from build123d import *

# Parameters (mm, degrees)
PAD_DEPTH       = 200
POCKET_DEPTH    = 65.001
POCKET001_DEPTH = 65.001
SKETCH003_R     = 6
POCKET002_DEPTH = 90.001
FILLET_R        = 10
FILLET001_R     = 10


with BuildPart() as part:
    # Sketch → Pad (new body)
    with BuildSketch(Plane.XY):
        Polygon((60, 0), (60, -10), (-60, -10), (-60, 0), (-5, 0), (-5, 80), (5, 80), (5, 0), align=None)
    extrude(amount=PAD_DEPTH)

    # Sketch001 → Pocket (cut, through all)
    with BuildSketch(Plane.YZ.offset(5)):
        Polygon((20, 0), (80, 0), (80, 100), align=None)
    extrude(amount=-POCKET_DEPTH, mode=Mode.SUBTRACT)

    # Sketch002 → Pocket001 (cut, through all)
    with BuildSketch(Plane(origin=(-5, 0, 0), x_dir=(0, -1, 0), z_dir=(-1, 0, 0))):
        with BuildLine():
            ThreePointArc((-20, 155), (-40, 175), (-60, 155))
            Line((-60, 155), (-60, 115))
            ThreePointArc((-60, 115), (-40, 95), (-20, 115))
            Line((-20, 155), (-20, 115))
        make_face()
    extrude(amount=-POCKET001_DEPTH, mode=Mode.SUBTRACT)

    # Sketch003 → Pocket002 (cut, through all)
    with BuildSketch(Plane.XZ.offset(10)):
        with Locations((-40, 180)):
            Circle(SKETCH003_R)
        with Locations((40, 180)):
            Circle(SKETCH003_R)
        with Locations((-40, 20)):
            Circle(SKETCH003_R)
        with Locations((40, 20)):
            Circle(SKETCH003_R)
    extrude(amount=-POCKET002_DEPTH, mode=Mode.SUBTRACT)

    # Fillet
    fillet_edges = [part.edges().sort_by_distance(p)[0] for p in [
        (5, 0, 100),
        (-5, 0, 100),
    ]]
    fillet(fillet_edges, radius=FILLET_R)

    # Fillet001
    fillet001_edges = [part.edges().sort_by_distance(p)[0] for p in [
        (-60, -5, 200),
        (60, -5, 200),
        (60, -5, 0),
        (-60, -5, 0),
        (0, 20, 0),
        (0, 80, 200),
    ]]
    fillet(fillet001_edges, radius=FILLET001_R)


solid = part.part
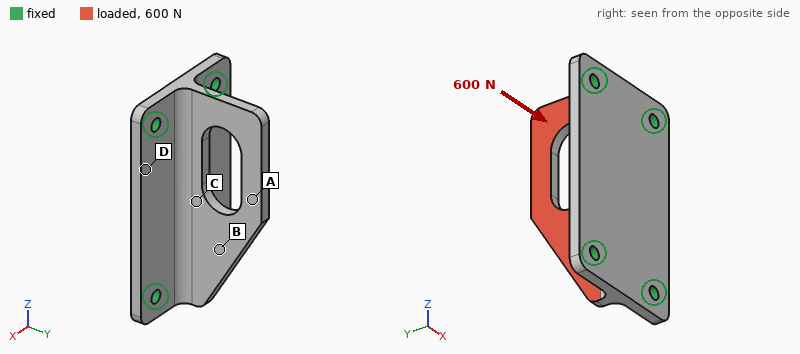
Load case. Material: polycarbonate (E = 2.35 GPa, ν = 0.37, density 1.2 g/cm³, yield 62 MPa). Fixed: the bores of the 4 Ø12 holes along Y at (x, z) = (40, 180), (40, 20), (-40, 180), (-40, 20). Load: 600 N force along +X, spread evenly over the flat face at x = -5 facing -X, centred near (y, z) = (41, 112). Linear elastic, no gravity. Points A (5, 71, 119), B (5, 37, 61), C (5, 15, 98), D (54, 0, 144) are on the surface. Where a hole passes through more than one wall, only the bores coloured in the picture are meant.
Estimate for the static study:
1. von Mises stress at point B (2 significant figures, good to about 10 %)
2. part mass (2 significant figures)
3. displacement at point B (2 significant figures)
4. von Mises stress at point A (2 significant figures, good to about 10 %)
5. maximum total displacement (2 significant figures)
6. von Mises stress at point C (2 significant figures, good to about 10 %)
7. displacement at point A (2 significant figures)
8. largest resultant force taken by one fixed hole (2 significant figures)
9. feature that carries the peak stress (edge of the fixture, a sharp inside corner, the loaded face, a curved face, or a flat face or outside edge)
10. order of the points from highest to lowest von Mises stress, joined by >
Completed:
4.5 MPa
410 g
0.48 mm
2.7 MPa
2.4 mm
6.4 MPa
1.9 mm
310 N
the loaded face
C > B > A > D
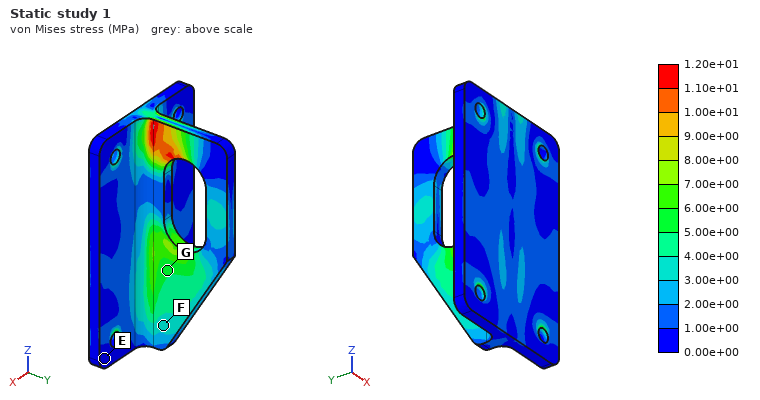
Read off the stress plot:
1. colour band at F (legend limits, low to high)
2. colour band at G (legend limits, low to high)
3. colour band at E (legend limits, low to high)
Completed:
3.00e+00 to 4.00e+00 MPa
5.00e+00 to 6.00e+00 MPa
0.00e+00 to 1.00e+00 MPa
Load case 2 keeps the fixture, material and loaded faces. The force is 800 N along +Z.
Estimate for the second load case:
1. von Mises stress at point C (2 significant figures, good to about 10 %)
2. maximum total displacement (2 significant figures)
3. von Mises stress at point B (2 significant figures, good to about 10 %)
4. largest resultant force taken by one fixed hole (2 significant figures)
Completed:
0.84 MPa
0.26 mm
0.78 MPa
260 N
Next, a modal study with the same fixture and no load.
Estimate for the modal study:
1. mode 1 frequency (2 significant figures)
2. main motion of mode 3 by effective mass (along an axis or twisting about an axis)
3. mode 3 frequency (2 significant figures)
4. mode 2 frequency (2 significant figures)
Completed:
320 Hz
along Y
740 Hz
590 Hz
